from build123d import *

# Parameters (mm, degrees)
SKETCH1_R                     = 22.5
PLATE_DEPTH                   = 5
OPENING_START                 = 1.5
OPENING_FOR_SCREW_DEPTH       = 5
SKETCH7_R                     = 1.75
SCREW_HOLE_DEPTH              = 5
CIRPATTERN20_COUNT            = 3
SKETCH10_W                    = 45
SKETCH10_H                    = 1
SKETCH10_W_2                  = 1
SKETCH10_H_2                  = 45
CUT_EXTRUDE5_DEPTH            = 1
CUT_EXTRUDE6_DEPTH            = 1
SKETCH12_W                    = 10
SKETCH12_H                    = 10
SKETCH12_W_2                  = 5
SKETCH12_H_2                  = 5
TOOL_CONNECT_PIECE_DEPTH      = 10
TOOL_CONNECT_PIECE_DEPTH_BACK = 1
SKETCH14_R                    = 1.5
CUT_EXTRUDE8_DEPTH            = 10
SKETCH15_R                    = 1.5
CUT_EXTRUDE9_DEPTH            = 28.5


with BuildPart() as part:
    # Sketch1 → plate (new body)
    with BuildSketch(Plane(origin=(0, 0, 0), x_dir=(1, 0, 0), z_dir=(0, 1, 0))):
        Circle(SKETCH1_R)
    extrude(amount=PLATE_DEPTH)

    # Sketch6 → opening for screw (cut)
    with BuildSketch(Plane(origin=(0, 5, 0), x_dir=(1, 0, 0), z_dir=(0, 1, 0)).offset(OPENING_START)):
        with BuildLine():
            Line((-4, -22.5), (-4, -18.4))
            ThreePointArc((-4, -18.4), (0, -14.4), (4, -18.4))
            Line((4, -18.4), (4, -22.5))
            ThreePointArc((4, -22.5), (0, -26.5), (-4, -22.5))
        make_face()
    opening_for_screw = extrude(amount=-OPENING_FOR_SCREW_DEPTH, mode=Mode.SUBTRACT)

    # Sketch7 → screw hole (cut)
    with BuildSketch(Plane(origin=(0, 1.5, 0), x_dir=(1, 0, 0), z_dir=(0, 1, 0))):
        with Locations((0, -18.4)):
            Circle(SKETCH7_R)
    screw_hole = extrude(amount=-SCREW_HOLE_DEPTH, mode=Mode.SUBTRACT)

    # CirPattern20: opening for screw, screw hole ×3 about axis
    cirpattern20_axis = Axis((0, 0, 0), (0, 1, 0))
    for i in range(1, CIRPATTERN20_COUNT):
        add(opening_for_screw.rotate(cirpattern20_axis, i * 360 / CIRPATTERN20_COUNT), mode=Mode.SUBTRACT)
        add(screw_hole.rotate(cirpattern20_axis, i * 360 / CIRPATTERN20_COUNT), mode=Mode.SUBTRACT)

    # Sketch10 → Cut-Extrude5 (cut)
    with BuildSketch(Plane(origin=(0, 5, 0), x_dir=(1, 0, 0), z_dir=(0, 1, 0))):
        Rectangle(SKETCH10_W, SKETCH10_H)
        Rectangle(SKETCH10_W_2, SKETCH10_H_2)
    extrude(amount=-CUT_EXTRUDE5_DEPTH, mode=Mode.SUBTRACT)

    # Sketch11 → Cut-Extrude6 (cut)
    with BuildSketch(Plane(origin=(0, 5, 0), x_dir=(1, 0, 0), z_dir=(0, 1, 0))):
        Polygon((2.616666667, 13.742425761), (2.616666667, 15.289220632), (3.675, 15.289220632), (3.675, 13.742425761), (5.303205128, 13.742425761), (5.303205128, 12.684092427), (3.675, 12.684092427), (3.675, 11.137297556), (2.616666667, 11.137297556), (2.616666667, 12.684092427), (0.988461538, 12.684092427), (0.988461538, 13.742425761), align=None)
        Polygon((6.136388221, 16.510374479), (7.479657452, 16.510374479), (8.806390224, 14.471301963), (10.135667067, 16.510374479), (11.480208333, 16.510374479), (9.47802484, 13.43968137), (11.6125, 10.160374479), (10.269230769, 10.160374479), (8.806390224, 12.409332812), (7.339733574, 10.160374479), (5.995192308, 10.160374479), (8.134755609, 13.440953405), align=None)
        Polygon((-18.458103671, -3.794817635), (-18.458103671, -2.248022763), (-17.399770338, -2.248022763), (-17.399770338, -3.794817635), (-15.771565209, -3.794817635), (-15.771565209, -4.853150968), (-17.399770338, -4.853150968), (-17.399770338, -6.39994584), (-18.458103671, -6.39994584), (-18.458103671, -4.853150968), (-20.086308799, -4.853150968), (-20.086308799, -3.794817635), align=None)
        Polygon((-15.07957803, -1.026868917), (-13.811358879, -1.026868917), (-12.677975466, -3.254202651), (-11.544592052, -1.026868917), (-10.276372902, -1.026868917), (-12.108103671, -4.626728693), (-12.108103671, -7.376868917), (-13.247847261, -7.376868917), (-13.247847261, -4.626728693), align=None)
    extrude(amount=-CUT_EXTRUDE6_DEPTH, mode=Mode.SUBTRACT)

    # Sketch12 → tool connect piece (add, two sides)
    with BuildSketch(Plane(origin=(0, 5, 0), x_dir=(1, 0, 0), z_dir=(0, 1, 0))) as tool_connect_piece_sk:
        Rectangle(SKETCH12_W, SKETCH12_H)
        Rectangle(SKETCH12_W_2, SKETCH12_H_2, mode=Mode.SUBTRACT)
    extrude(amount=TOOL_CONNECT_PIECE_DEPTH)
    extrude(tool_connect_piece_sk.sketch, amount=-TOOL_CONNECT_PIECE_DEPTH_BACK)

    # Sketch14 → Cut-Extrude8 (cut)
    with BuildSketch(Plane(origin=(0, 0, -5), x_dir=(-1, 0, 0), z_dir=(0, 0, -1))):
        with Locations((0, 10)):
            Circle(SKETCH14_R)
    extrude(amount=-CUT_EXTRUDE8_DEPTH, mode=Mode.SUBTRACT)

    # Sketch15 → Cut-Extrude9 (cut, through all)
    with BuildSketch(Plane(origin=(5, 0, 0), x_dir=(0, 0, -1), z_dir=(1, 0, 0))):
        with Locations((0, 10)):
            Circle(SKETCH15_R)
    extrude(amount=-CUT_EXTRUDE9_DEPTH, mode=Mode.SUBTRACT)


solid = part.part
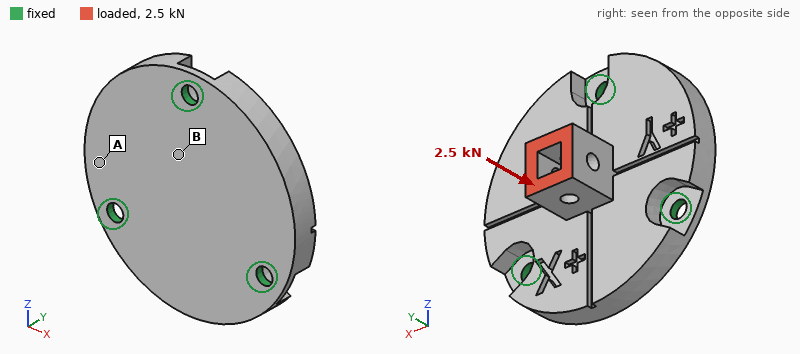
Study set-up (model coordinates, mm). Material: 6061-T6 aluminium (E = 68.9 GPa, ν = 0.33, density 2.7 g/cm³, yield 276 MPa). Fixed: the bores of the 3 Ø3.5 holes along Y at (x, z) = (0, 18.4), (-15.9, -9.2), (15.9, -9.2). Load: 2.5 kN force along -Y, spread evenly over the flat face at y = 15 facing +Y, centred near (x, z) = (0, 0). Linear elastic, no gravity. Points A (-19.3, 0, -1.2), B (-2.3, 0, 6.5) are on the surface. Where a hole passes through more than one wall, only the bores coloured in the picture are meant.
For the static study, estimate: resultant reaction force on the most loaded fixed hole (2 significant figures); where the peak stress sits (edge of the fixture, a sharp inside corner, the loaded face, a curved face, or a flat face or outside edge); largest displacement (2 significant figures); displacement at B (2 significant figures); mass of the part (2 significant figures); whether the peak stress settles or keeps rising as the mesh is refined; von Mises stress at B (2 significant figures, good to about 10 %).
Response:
1.2 kN
edge of the fixture
48 µm
38 µm
21 g
keeps rising
48 MPa
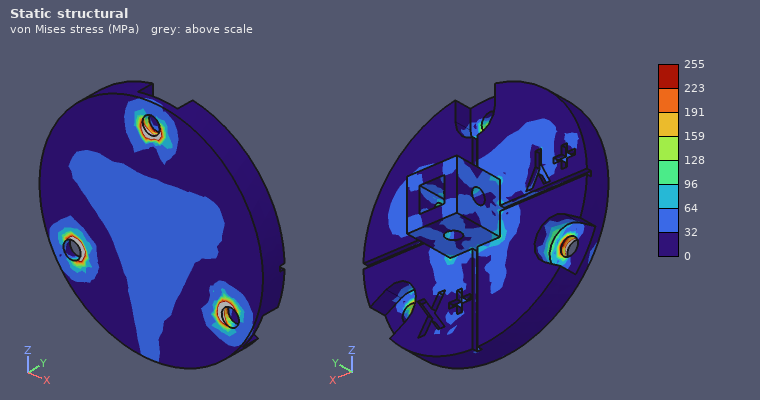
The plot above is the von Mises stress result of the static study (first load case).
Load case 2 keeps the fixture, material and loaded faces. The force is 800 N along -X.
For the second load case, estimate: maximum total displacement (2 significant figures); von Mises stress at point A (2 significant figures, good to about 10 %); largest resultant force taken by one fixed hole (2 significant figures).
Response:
44 µm
8.9 MPa
600 N
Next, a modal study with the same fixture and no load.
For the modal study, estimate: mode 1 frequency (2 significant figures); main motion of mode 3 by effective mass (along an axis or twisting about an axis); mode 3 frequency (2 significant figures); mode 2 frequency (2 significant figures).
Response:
9900 Hz
along Y
11 kHz
10000 Hz
